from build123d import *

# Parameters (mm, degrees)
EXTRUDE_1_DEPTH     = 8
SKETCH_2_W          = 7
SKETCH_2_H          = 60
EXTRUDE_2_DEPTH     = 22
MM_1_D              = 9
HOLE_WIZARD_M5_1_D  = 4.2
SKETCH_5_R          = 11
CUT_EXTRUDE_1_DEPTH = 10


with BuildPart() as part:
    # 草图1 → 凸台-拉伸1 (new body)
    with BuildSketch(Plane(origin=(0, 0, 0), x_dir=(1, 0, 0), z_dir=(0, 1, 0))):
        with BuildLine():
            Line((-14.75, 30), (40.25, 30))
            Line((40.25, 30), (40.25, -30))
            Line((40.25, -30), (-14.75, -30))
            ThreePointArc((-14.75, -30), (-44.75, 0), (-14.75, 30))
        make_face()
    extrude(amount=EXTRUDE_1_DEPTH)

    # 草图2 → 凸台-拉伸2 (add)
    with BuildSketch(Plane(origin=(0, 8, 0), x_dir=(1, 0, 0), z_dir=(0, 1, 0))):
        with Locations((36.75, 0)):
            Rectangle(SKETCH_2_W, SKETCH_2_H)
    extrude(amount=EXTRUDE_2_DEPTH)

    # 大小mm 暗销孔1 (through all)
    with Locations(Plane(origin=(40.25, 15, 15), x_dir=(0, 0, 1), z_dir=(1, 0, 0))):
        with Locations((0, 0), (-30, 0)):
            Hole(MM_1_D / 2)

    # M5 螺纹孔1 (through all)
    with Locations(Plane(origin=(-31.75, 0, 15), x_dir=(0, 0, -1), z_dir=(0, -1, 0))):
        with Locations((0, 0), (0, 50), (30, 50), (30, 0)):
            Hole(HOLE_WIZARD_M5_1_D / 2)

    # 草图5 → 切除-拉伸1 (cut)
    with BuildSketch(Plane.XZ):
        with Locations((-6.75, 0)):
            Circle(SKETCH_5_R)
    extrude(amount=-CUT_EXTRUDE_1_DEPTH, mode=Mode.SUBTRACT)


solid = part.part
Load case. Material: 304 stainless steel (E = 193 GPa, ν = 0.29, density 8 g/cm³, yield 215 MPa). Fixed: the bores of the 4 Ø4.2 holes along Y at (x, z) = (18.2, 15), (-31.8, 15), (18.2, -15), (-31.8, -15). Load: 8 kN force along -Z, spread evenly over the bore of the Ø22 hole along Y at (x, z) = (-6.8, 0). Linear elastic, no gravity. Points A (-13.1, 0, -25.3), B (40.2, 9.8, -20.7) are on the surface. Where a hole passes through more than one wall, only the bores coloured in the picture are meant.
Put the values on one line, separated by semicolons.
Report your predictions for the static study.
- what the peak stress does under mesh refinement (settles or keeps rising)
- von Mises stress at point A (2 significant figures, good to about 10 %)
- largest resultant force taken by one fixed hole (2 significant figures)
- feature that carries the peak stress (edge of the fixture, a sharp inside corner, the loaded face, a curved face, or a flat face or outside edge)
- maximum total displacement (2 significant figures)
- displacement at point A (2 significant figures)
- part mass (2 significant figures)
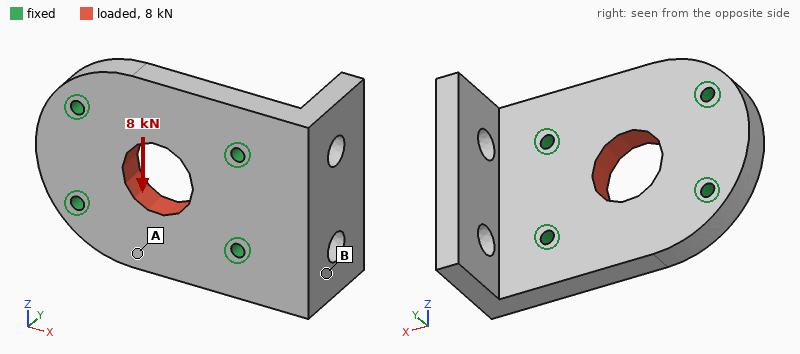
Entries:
keeps rising; 12 MPa; 2.2 kN; edge of the fixture; 3.6 µm; 2.7 µm; 340 g
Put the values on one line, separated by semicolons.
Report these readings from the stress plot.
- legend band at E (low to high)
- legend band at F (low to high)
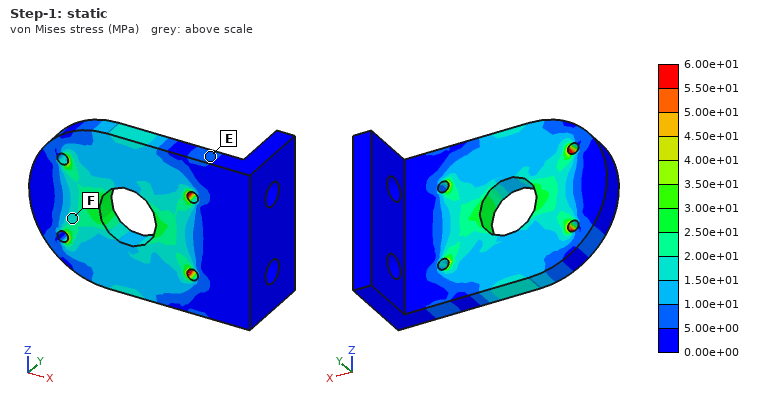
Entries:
5.00e+00 to 1.00e+01 MPa; 1.50e+01 to 2.00e+01 MPa
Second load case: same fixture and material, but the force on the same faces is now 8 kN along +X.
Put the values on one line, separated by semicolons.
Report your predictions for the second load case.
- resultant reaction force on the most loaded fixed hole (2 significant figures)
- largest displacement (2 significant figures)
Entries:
2.1 kN; 1.8 µm
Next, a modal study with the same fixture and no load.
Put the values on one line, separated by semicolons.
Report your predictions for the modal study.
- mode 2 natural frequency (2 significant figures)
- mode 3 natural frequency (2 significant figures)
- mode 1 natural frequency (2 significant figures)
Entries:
6200 Hz; 9700 Hz; 4100 Hz
